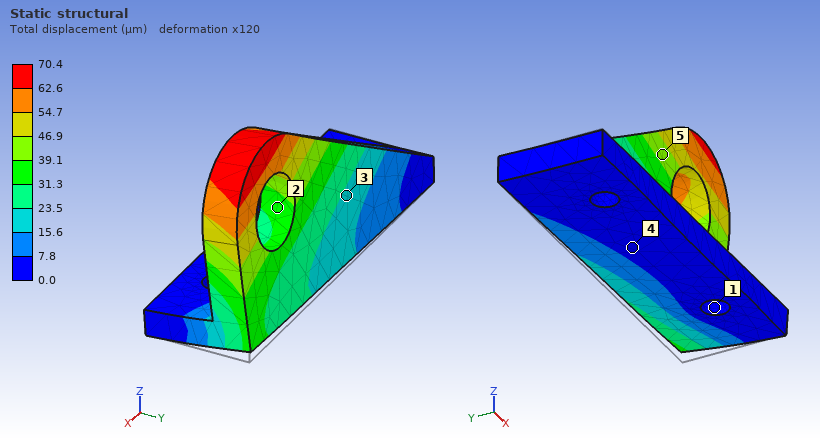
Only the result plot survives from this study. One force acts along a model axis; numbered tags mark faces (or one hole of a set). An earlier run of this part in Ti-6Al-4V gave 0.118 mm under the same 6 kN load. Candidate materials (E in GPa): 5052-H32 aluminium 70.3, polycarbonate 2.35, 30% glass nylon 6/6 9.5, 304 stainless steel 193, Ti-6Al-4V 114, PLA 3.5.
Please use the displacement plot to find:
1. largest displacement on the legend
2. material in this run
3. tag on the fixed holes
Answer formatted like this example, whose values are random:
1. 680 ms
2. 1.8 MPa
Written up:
1. 70.4 µm
2. 304 stainless steel
3. 1
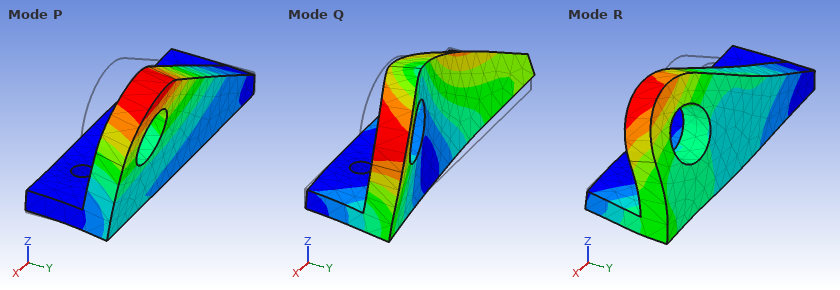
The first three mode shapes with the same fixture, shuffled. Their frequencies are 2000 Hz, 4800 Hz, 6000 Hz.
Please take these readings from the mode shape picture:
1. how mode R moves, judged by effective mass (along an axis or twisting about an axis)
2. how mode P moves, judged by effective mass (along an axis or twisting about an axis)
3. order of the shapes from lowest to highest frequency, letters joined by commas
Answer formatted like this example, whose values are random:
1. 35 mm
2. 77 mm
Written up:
1. along Z
2. along Y
3. P, Q, R
